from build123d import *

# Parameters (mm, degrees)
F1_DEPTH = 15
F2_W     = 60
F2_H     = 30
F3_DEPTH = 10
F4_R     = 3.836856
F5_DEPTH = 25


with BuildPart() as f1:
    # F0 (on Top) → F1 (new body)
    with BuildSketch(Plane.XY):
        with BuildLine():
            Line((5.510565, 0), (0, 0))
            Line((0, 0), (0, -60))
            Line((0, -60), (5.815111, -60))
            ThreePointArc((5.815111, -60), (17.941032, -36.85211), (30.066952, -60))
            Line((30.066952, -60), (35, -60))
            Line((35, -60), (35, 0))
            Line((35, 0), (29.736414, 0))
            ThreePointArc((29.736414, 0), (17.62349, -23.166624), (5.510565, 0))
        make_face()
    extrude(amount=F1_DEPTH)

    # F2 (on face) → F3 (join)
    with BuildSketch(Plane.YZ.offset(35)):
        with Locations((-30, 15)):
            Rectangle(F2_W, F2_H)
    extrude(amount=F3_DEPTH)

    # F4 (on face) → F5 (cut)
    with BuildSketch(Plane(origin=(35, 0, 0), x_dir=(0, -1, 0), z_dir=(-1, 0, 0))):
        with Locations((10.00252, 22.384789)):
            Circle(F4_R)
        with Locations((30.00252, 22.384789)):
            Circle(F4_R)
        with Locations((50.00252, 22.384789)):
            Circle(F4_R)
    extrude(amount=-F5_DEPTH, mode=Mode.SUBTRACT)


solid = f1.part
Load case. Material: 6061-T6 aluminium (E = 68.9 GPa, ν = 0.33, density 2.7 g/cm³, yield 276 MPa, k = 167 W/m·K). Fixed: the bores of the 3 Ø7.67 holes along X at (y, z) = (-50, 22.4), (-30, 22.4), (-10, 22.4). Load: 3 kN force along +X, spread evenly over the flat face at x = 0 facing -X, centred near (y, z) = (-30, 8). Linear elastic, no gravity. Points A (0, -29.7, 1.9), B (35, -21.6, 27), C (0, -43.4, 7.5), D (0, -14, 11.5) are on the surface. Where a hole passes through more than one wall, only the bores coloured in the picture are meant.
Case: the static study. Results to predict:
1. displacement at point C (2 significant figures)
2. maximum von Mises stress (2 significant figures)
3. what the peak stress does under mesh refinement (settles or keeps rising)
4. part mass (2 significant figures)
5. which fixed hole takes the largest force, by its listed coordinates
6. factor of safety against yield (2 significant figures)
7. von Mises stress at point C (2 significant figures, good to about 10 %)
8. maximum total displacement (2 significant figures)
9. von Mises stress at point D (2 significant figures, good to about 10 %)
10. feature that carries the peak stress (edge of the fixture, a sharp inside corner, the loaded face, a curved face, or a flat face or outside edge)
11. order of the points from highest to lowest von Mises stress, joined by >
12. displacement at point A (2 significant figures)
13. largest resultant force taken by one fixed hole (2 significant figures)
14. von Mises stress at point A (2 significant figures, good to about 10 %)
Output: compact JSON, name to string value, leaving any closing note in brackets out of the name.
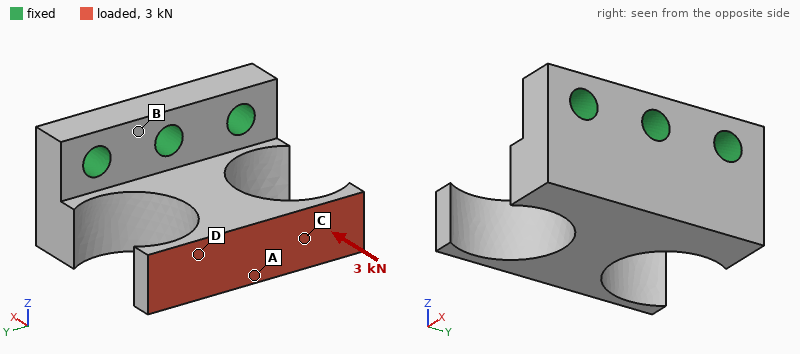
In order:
{"displacement at point C": "0.046 mm", "maximum von Mises stress": "140 MPa", "what the peak stress does under mesh refinement": "settles", "part mass": "83 g", "which fixed hole takes the largest force, by its listed coordinates": "(-30, 22.4)", "factor of safety against yield": "2.0", "von Mises stress at point C": "94 MPa", "maximum total displacement": "0.20 mm", "von Mises stress at point D": "120 MPa", "feature that carries the peak stress": "a curved face", "order of the points from highest to lowest von Mises stress, joined by >": "D > C > A > B", "displacement at point A": "0.040 mm", "largest resultant force taken by one fixed hole": "1.5 kN", "von Mises stress at point A": "38 MPa"}
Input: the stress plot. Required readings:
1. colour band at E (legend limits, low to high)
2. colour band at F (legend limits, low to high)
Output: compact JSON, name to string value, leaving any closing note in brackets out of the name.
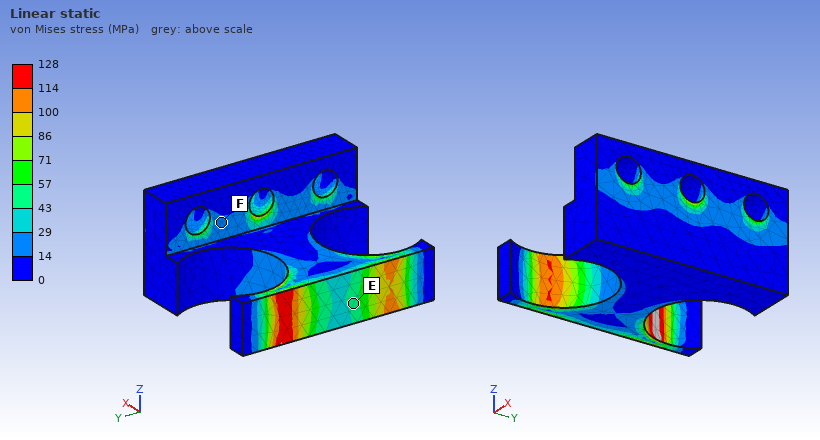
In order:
{"colour band at E": "43 to 57 MPa", "colour band at F": "14 to 29 MPa"}
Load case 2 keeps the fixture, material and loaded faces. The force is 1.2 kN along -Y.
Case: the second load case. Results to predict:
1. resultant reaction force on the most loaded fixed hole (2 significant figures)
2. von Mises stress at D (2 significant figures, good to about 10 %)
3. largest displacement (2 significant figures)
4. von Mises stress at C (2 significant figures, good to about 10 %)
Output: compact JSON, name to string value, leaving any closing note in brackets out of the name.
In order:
{"resultant reaction force on the most loaded fixed hole": "1.2 kN", "von Mises stress at D": "19 MPa", "largest displacement": "0.11 mm", "von Mises stress at C": "17 MPa"}
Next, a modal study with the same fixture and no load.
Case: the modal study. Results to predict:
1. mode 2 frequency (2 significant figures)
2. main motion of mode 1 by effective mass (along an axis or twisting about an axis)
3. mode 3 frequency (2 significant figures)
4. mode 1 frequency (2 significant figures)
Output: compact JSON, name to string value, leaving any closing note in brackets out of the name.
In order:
{"mode 2 frequency": "5200 Hz", "main motion of mode 1 by effective mass": "along Z", "mode 3 frequency": "7200 Hz", "mode 1 frequency": "3900 Hz"}
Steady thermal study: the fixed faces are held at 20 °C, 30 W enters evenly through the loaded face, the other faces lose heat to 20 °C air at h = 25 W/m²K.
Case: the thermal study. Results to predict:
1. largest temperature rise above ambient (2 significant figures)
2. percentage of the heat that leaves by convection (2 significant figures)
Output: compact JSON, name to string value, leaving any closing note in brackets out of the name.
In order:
{"largest temperature rise above ambient": "36 K", "percentage of the heat that leaves by convection": "6.2 %"}
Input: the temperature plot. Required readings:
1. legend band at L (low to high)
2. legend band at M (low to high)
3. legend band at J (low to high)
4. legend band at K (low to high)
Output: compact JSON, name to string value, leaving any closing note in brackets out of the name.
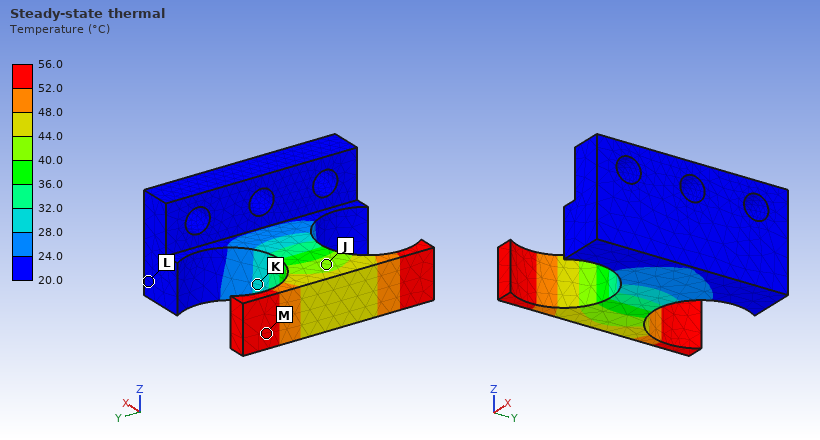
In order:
{"legend band at L": "20.0 to 24.0 °C", "legend band at M": "52.0 to 56.0 °C", "legend band at J": "40.0 to 44.0 °C", "legend band at K": "28.0 to 32.0 °C"}
